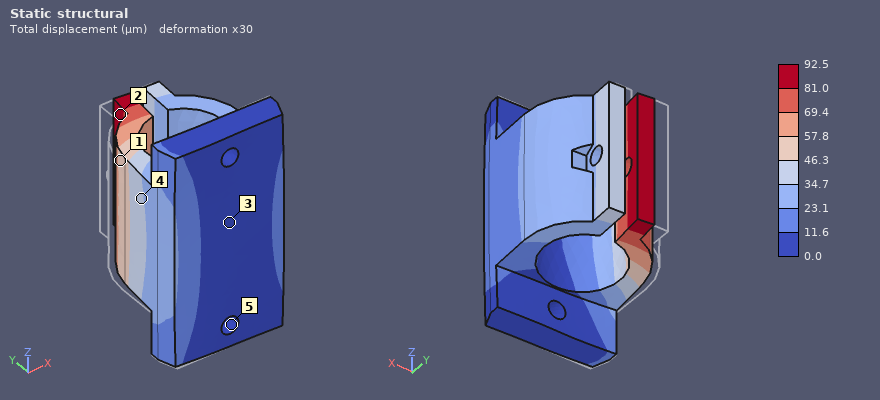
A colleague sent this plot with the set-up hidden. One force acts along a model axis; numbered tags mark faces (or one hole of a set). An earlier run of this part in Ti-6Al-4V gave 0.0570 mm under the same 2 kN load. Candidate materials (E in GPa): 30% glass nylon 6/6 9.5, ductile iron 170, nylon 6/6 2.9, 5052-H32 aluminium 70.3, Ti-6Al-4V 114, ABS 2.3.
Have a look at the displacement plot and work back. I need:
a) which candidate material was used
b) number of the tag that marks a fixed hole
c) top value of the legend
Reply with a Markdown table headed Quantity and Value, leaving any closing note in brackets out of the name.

| Quantity | Value |
|---|---|
| which candidate material was used | 5052-H32 aluminium |
| number of the tag that marks a fixed hole | 5 |
| top value of the legend | 92.5 µm |
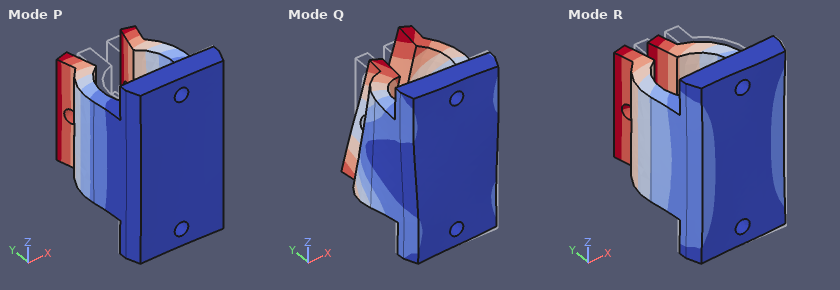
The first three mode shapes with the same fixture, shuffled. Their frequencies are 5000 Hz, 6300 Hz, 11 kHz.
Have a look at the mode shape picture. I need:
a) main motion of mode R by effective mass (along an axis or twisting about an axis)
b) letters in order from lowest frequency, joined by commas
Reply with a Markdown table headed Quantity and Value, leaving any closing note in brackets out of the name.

| Quantity | Value |
|---|---|
| main motion of mode R by effective mass | along X |
| letters in order from lowest frequency, joined by commas | R, P, Q |
